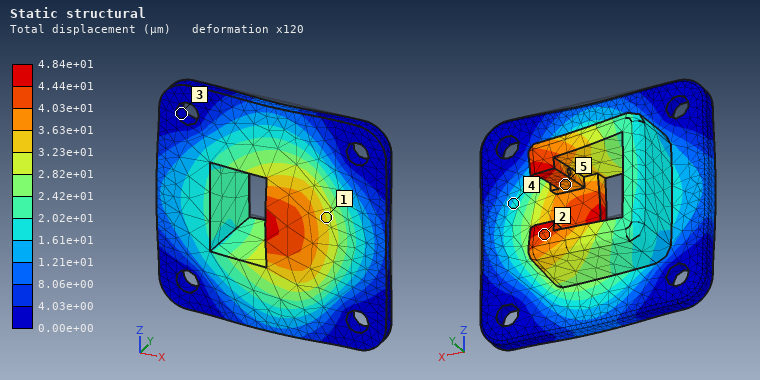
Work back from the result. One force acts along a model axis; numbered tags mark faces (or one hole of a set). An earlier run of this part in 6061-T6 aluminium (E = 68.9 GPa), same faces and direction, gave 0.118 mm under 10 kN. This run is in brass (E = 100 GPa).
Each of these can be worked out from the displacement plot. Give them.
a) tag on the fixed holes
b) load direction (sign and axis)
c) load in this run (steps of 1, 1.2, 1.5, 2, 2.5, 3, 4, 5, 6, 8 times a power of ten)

3
-Y
6 kN
